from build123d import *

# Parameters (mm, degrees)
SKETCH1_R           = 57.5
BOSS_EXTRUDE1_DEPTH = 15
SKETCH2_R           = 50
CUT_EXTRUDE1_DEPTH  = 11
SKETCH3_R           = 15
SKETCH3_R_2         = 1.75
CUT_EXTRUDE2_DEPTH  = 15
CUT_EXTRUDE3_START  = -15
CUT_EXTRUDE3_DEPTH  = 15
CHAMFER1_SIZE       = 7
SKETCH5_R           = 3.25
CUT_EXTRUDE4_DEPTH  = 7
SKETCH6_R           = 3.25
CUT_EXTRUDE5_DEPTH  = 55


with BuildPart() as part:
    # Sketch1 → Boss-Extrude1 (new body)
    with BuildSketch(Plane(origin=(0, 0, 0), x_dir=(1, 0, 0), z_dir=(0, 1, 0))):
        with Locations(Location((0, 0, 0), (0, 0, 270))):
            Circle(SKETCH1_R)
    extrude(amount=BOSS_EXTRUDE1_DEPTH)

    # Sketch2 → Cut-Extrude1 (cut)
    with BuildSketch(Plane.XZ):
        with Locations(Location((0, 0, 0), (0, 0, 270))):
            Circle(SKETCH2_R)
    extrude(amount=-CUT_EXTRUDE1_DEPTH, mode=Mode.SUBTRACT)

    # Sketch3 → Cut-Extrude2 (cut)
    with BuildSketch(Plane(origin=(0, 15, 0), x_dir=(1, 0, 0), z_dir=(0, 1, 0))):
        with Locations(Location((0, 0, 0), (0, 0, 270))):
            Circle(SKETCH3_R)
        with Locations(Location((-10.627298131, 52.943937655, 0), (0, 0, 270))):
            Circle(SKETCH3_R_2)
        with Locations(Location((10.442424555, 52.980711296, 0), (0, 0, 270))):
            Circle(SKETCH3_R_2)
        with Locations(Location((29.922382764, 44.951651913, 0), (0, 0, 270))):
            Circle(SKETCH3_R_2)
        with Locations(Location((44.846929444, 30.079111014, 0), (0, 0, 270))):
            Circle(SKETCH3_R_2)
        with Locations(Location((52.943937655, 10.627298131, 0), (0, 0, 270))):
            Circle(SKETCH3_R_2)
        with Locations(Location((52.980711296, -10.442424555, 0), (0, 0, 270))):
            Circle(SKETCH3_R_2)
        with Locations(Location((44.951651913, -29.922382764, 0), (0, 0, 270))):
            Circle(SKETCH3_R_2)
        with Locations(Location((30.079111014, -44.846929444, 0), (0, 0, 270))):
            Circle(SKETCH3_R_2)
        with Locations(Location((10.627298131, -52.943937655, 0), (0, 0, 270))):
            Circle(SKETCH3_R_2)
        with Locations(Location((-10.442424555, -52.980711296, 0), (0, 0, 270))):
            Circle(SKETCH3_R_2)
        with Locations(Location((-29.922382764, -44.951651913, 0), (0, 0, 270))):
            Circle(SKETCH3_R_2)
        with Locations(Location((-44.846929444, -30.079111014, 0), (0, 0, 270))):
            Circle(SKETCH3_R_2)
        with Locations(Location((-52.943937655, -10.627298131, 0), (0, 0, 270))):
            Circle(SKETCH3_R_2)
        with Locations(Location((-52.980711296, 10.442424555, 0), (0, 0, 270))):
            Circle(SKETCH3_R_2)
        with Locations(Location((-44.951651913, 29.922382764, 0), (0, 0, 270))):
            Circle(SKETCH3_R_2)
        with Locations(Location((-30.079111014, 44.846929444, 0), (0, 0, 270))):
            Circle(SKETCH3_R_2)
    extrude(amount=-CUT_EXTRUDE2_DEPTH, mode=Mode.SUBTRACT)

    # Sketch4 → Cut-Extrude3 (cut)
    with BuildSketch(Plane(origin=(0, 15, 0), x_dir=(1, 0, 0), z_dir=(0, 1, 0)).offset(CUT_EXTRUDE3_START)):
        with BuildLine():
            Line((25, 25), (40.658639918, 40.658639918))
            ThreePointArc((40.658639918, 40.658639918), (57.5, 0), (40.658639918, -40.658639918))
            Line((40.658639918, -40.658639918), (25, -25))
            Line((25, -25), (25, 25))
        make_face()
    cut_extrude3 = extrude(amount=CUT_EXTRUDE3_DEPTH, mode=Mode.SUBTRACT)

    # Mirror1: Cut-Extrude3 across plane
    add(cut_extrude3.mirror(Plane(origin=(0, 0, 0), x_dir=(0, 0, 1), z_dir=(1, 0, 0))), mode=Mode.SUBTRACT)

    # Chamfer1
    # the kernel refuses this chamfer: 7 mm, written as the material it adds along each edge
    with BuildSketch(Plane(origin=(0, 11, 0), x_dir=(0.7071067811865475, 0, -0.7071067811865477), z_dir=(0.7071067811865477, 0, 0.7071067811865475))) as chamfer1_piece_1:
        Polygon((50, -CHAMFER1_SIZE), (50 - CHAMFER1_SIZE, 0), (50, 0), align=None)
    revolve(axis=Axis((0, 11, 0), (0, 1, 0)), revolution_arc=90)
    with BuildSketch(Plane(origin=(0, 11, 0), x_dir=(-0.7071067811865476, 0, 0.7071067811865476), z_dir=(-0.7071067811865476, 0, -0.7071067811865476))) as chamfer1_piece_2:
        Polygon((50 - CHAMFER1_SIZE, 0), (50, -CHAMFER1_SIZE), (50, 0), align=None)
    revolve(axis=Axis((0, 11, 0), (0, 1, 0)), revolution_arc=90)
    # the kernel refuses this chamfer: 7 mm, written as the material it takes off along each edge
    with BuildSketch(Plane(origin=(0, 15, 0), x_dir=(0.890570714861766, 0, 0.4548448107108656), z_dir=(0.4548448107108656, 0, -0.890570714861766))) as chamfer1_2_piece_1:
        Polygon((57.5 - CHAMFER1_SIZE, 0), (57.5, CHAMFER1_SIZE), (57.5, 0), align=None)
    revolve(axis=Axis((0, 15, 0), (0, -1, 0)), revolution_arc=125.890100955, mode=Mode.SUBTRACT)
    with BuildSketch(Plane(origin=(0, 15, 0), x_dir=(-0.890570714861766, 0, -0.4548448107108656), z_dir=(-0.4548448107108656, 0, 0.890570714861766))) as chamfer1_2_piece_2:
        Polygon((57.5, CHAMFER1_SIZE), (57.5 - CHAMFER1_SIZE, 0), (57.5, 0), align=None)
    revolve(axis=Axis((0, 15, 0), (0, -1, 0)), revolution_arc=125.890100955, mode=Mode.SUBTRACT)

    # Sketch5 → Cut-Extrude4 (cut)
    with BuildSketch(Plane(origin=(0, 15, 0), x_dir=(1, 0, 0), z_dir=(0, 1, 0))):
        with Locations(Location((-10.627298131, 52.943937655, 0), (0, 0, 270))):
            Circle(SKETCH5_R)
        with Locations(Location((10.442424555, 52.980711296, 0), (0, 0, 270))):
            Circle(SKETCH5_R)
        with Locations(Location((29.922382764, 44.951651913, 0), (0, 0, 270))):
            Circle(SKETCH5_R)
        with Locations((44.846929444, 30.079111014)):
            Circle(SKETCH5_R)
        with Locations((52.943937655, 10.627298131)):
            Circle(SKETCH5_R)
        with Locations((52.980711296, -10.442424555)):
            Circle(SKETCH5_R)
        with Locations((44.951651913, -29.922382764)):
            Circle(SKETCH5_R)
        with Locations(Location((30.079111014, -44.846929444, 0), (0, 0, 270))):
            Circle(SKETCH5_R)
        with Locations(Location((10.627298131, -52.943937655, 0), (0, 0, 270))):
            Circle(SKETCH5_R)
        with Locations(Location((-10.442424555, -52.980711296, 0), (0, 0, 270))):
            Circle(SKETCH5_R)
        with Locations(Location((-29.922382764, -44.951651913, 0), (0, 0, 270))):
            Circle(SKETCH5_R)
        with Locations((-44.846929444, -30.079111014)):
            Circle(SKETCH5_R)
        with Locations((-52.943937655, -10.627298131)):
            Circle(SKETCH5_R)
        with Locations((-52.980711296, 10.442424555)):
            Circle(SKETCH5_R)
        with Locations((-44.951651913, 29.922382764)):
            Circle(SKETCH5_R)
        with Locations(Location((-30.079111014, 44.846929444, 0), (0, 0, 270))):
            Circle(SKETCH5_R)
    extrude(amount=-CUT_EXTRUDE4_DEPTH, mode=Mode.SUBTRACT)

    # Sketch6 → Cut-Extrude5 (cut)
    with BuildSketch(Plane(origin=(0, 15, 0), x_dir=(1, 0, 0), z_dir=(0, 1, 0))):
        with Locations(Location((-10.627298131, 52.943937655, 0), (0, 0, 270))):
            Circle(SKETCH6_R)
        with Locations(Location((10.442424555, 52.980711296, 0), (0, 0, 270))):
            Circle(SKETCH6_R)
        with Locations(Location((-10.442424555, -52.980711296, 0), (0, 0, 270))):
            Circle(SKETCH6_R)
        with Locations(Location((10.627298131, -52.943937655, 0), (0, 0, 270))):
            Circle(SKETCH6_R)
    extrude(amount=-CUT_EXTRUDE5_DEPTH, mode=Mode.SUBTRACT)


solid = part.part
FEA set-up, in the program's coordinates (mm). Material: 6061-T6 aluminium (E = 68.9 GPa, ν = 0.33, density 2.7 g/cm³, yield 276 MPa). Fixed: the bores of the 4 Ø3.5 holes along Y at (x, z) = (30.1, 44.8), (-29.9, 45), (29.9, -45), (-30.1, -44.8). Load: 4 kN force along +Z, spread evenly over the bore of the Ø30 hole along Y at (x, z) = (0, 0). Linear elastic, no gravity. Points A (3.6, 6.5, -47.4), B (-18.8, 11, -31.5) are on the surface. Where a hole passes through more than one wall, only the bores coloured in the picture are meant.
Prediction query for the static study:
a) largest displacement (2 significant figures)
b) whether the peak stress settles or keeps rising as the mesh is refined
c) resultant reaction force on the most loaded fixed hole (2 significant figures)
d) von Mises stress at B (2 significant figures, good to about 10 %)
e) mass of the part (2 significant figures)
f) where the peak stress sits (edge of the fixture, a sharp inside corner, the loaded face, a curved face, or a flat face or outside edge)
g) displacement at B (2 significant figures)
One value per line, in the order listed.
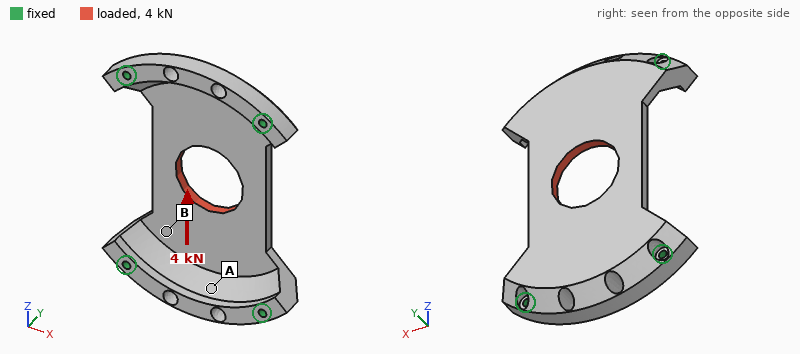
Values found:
27 µm
keeps rising
1.0 kN
22 MPa
92 g
edge of the fixture
22 µm
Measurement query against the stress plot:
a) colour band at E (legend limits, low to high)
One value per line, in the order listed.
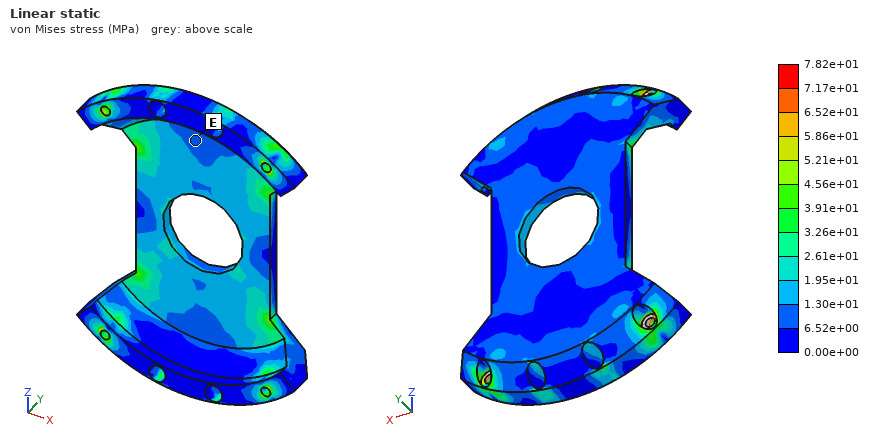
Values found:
6.52e+00 to 1.30e+01 MPa
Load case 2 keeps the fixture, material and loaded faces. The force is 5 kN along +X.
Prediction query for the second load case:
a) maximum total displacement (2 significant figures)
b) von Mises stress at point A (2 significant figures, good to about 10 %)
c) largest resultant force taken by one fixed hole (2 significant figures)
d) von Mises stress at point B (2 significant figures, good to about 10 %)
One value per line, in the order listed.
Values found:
45 µm
14 MPa
1.5 kN
27 MPa
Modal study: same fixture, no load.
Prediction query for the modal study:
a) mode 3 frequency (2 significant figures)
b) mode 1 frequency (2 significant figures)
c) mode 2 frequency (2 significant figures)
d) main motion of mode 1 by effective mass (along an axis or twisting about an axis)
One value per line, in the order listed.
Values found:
6000 Hz
3400 Hz
4900 Hz
along Y
